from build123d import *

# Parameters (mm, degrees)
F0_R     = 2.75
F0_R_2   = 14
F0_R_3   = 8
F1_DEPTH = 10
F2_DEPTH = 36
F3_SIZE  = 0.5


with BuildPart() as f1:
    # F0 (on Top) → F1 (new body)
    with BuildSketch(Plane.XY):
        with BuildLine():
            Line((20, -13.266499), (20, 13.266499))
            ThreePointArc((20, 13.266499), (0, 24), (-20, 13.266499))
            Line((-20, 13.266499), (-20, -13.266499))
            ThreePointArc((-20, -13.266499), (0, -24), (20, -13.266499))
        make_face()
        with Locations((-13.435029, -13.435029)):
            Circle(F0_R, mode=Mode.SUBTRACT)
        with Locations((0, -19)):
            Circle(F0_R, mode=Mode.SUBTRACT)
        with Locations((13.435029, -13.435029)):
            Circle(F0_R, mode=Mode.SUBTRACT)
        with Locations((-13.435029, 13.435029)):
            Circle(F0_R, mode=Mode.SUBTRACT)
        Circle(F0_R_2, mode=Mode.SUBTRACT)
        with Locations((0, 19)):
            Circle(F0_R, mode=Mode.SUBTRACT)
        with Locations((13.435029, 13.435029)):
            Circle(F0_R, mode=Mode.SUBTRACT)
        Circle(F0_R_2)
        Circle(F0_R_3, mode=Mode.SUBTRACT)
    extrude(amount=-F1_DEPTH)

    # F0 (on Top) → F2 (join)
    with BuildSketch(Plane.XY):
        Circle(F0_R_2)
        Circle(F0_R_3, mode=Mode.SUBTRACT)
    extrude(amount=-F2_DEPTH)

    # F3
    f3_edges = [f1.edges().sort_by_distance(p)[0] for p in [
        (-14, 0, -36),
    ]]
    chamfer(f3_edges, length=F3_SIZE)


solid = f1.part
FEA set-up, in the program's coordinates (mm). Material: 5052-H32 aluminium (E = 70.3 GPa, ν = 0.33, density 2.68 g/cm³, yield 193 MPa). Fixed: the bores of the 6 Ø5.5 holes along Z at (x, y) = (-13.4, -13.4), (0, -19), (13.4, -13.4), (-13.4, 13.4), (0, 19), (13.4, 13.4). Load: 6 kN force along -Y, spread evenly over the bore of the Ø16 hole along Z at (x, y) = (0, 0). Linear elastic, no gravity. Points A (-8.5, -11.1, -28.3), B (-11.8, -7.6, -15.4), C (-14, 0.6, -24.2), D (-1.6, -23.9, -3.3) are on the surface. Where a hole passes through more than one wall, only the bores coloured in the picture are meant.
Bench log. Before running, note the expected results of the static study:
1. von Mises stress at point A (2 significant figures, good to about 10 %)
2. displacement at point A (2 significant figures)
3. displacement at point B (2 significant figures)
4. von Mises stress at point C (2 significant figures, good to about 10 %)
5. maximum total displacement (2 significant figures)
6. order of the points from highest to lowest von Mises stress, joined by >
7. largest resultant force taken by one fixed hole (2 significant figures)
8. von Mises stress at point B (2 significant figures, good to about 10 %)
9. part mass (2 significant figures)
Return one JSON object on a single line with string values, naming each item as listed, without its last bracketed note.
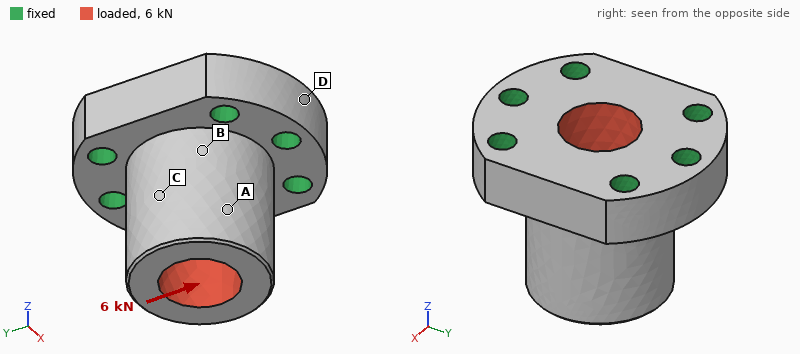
{"von Mises stress at point A": "6.7 MPa", "displacement at point A": "16 µm", "displacement at point B": "6.0 µm", "von Mises stress at point C": "12 MPa", "maximum total displacement": "21 µm", "order of the points from highest to lowest von Mises stress, joined by >": "B > C > A > D", "largest resultant force taken by one fixed hole": "1.7 kN", "von Mises stress at point B": "17 MPa", "part mass": "64 g"}
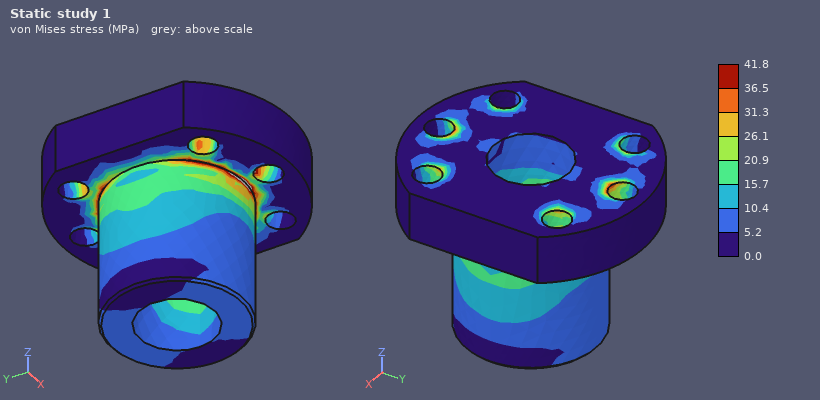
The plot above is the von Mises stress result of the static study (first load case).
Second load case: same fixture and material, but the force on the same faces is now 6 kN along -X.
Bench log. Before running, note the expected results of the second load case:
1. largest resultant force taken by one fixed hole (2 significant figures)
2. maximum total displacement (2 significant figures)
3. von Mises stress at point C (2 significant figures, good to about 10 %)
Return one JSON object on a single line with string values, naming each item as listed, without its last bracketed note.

{"largest resultant force taken by one fixed hole": "1.9 kN", "maximum total displacement": "25 µm", "von Mises stress at point C": "7.1 MPa"}
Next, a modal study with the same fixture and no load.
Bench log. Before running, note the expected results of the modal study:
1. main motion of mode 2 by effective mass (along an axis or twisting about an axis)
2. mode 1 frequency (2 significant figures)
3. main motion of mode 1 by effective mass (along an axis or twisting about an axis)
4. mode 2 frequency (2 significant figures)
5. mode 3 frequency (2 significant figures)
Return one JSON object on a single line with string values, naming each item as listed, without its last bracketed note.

{"main motion of mode 2 by effective mass": "along Y", "mode 1 frequency": "15 kHz", "main motion of mode 1 by effective mass": "along X", "mode 2 frequency": "16 kHz", "mode 3 frequency": "27 kHz"}
